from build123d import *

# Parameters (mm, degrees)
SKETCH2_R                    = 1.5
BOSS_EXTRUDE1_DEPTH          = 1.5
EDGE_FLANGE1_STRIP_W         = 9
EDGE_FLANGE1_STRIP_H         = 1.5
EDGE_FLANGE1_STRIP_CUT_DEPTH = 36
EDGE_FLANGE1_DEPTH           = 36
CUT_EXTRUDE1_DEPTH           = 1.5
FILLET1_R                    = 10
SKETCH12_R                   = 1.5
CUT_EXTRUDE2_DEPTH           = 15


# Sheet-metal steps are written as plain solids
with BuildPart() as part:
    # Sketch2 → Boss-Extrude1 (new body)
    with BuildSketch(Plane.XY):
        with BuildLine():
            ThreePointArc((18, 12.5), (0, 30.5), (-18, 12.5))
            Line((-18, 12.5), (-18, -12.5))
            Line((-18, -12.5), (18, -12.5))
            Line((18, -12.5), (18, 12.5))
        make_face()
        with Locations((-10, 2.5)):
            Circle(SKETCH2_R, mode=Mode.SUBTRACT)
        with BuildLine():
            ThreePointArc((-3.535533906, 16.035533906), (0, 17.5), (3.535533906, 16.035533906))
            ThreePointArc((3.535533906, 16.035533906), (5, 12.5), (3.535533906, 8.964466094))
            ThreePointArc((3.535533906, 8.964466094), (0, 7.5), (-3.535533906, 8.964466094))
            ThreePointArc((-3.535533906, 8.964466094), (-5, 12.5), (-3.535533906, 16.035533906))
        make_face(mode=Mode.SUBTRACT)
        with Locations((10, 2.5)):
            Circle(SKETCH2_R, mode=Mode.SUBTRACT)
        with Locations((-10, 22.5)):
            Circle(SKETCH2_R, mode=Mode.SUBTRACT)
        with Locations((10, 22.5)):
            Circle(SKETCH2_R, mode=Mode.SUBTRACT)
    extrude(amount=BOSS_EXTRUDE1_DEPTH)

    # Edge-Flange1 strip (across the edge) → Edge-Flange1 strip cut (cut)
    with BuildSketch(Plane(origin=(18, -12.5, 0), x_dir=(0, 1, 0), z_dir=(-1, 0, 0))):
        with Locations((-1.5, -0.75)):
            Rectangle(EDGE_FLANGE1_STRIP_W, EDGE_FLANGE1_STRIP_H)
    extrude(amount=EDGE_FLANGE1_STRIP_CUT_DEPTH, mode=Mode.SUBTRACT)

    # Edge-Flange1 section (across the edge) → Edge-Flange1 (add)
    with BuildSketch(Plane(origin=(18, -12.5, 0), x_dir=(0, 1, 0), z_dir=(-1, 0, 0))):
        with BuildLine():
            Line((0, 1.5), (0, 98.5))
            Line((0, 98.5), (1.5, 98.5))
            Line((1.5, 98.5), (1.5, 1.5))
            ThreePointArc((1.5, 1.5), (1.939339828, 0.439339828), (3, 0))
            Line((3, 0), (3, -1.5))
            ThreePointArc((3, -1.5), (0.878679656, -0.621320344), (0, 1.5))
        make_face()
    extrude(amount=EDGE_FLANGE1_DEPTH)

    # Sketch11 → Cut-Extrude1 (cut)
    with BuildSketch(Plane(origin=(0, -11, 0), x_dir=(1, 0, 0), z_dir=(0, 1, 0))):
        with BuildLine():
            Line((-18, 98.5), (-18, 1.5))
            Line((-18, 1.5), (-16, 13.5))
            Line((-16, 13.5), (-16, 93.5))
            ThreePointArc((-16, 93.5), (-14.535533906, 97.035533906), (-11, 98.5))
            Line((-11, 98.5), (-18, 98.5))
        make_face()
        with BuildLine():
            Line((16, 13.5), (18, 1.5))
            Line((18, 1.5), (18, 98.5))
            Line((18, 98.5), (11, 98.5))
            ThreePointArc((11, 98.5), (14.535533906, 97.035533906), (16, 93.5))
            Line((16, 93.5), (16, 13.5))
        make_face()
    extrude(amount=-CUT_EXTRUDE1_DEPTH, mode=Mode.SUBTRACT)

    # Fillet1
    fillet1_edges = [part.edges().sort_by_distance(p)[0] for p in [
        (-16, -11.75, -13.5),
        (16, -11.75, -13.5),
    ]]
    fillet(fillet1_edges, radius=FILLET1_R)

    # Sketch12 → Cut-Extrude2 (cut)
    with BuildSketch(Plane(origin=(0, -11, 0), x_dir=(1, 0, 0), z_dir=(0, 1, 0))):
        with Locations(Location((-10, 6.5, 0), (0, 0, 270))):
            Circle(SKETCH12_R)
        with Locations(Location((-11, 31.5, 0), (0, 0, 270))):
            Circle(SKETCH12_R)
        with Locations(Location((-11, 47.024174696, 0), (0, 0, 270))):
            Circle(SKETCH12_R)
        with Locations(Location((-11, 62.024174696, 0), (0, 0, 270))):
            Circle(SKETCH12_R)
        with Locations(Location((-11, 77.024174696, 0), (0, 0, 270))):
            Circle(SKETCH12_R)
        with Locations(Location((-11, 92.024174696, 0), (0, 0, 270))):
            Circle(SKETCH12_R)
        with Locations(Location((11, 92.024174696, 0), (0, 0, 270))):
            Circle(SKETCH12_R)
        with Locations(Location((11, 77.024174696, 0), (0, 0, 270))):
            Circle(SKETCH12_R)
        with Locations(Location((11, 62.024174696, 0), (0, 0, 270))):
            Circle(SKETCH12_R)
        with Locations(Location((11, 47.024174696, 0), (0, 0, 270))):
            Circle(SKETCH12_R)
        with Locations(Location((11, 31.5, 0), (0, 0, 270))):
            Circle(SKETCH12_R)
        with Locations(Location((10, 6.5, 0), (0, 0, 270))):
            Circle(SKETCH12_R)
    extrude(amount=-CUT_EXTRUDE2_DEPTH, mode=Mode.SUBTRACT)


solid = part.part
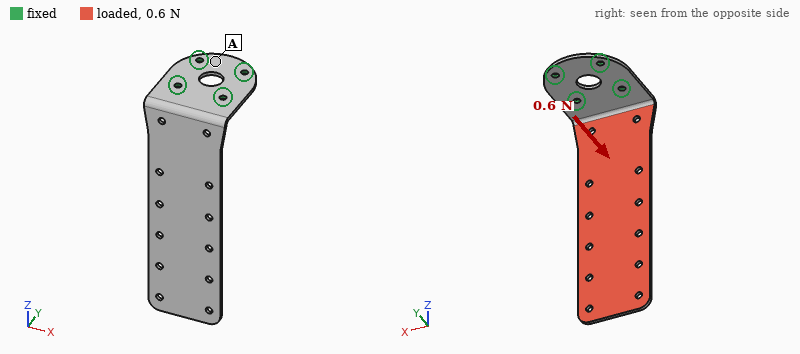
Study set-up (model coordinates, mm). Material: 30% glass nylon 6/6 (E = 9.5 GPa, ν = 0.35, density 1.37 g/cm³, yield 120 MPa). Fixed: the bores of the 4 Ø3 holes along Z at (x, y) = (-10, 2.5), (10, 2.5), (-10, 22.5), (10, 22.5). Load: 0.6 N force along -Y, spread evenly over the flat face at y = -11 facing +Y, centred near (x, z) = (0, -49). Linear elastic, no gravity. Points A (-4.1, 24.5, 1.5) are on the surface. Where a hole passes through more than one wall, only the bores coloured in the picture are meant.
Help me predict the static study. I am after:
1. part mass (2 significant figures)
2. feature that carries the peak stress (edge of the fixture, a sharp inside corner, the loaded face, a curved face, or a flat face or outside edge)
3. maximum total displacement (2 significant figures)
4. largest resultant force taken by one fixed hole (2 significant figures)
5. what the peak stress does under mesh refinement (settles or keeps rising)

8.9 g
edge of the fixture
1.2 mm
0.40 N
keeps rising
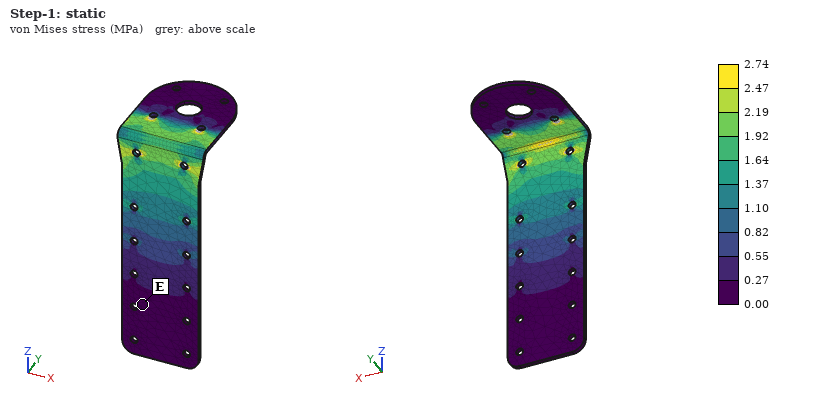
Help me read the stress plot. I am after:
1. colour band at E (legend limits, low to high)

0.00 to 0.27 MPa
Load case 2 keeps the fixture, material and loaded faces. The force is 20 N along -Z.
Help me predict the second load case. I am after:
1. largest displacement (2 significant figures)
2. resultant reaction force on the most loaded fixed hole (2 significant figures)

1.2 mm
11 N
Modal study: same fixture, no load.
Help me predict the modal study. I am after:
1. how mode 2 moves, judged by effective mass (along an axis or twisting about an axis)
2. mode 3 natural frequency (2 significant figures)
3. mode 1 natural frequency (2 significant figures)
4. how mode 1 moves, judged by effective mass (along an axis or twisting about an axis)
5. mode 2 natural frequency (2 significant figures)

along X
350 Hz
56 Hz
along Y
190 Hz
